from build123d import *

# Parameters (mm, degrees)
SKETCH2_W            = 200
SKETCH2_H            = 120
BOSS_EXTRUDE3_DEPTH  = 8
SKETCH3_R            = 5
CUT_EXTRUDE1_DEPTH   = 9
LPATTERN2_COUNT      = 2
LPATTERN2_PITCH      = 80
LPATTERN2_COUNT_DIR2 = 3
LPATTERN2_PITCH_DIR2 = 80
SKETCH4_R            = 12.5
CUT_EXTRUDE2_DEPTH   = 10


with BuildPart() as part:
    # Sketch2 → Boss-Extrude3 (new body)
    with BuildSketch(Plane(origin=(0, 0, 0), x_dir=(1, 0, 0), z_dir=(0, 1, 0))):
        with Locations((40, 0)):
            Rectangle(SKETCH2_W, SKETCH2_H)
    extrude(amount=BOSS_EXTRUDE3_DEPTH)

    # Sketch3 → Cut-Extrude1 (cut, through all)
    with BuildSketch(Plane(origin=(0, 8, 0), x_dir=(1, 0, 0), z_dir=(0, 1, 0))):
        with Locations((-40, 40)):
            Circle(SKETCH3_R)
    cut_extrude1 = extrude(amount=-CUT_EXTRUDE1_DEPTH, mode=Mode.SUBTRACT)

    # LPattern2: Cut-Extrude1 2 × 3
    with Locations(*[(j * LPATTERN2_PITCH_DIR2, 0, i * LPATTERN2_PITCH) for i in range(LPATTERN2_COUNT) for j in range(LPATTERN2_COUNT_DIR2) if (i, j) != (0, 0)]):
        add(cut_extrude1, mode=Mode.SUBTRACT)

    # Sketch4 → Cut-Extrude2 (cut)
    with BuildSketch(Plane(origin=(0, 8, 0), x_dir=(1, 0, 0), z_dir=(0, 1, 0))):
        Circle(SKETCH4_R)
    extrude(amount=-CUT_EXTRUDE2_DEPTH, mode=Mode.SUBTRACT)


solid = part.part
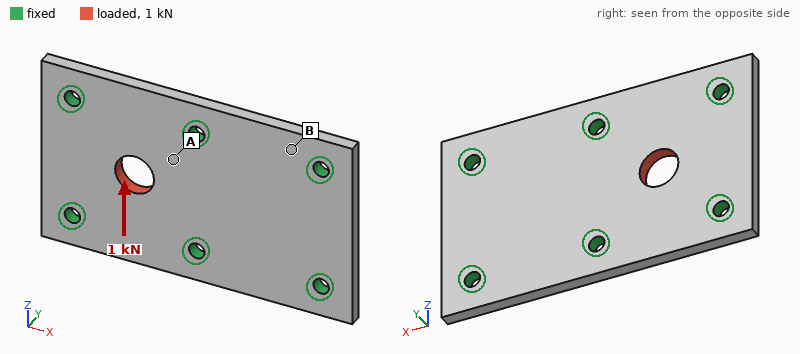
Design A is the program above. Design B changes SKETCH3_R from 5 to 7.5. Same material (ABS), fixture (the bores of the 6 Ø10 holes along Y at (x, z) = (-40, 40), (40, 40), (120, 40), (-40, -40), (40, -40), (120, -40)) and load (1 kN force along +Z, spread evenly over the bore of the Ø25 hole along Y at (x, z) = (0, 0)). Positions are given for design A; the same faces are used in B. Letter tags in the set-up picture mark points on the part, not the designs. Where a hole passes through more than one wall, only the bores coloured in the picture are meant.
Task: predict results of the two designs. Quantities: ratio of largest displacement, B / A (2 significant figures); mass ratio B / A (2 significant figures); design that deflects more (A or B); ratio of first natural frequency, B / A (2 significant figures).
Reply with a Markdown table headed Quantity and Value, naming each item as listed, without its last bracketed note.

| Quantity | Value |
|---|---|
| ratio of largest displacement, B / A | 0.91 |
| mass ratio B / A | 0.97 |
| design that deflects more | A |
| ratio of first natural frequency, B / A | 1.1 |
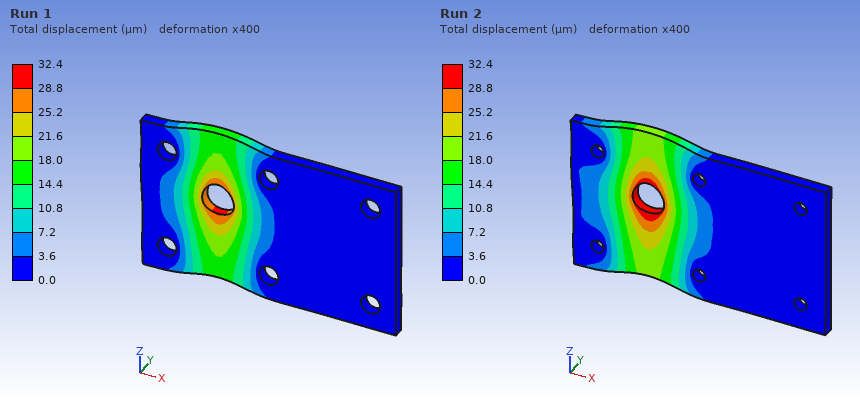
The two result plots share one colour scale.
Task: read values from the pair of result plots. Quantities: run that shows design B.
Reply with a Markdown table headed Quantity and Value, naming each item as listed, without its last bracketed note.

| Quantity | Value |
|---|---|
| run that shows design B | Run 1 |
